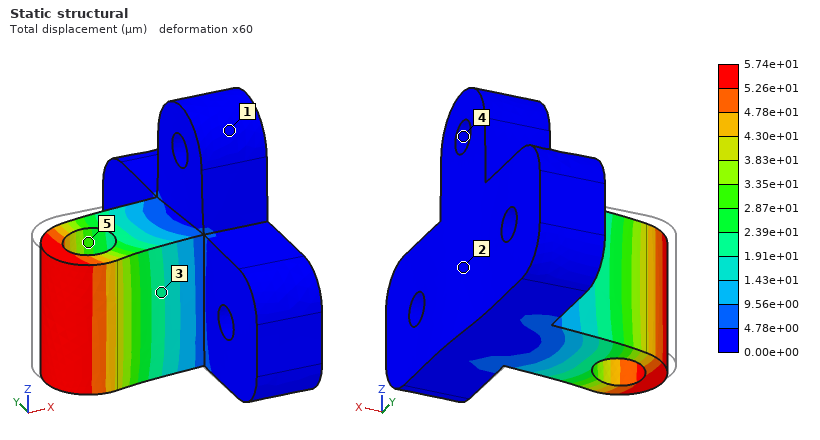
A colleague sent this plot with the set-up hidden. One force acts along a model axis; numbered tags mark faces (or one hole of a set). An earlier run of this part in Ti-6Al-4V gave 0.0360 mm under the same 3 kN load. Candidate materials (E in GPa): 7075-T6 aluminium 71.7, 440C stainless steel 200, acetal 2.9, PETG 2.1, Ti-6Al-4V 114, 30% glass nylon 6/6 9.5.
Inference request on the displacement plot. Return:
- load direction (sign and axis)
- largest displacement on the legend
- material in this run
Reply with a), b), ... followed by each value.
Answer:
a) -Y
b) 5.74e+01 µm
c) 7075-T6 aluminium
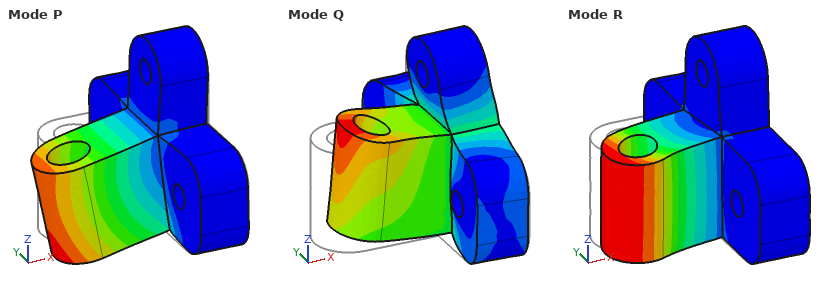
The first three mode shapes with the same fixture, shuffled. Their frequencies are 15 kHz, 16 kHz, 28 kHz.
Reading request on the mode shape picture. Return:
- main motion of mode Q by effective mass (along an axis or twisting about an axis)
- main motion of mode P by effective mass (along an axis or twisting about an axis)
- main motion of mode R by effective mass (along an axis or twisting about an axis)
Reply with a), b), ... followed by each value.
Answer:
a) along X
b) along Z
c) along Y
